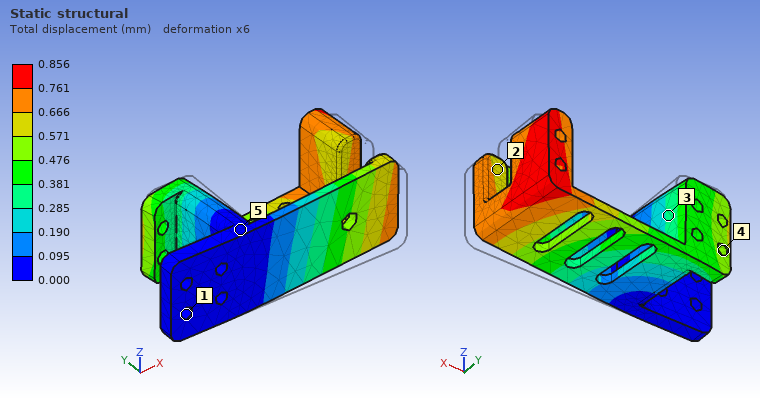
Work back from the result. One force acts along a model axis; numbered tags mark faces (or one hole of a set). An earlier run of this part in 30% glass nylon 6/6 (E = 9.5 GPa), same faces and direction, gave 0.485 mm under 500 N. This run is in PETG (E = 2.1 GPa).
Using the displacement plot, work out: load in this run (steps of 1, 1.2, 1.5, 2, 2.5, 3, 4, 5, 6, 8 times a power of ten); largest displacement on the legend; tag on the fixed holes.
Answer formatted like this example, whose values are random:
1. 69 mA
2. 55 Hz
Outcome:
1. 200 N
2. 0.856 mm
3. 1
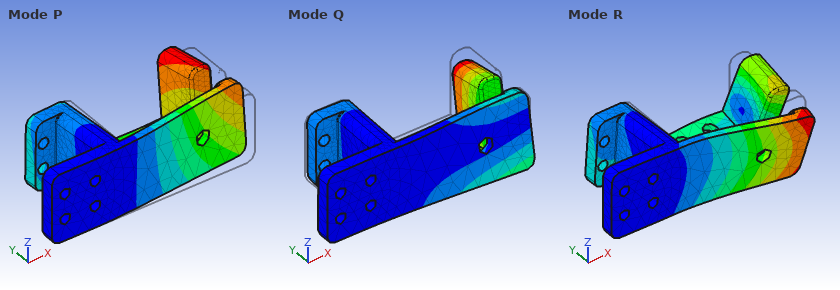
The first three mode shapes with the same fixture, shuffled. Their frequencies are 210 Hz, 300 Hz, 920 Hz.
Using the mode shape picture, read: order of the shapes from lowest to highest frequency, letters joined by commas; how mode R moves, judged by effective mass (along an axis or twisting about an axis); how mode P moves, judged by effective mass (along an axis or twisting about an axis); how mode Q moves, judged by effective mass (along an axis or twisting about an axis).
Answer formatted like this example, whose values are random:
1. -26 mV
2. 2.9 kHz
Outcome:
1. P, Q, R
2. along Z
3. along Y
4. along Z
